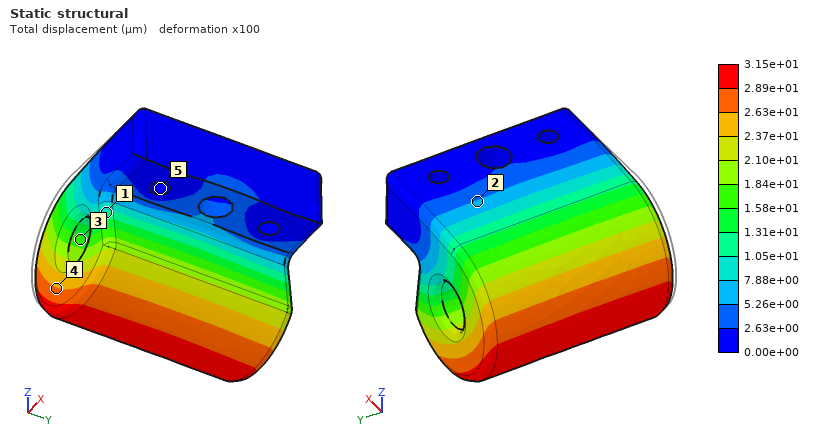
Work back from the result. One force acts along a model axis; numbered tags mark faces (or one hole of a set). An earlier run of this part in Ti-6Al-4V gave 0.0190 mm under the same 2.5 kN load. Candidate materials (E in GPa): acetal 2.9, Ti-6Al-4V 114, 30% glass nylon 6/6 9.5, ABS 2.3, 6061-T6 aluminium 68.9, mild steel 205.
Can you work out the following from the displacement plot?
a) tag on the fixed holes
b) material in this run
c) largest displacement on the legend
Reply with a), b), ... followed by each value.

a) 5
b) 6061-T6 aluminium
c) 3.15e+01 µm
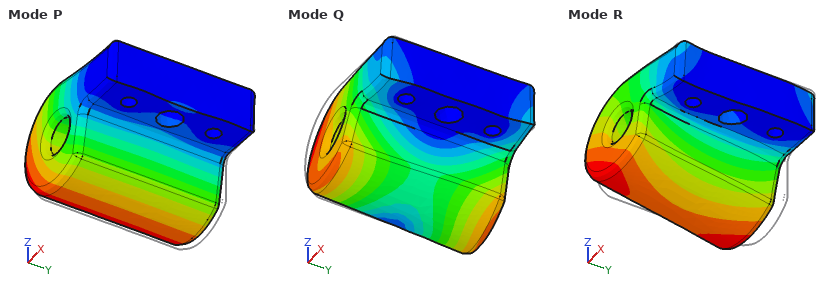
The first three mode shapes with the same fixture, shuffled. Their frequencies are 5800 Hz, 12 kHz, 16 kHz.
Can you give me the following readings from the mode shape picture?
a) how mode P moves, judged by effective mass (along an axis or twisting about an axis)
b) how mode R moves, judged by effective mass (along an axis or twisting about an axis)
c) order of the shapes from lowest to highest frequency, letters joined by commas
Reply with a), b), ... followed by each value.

a) along Z
b) along Y
c) P, R, Q
